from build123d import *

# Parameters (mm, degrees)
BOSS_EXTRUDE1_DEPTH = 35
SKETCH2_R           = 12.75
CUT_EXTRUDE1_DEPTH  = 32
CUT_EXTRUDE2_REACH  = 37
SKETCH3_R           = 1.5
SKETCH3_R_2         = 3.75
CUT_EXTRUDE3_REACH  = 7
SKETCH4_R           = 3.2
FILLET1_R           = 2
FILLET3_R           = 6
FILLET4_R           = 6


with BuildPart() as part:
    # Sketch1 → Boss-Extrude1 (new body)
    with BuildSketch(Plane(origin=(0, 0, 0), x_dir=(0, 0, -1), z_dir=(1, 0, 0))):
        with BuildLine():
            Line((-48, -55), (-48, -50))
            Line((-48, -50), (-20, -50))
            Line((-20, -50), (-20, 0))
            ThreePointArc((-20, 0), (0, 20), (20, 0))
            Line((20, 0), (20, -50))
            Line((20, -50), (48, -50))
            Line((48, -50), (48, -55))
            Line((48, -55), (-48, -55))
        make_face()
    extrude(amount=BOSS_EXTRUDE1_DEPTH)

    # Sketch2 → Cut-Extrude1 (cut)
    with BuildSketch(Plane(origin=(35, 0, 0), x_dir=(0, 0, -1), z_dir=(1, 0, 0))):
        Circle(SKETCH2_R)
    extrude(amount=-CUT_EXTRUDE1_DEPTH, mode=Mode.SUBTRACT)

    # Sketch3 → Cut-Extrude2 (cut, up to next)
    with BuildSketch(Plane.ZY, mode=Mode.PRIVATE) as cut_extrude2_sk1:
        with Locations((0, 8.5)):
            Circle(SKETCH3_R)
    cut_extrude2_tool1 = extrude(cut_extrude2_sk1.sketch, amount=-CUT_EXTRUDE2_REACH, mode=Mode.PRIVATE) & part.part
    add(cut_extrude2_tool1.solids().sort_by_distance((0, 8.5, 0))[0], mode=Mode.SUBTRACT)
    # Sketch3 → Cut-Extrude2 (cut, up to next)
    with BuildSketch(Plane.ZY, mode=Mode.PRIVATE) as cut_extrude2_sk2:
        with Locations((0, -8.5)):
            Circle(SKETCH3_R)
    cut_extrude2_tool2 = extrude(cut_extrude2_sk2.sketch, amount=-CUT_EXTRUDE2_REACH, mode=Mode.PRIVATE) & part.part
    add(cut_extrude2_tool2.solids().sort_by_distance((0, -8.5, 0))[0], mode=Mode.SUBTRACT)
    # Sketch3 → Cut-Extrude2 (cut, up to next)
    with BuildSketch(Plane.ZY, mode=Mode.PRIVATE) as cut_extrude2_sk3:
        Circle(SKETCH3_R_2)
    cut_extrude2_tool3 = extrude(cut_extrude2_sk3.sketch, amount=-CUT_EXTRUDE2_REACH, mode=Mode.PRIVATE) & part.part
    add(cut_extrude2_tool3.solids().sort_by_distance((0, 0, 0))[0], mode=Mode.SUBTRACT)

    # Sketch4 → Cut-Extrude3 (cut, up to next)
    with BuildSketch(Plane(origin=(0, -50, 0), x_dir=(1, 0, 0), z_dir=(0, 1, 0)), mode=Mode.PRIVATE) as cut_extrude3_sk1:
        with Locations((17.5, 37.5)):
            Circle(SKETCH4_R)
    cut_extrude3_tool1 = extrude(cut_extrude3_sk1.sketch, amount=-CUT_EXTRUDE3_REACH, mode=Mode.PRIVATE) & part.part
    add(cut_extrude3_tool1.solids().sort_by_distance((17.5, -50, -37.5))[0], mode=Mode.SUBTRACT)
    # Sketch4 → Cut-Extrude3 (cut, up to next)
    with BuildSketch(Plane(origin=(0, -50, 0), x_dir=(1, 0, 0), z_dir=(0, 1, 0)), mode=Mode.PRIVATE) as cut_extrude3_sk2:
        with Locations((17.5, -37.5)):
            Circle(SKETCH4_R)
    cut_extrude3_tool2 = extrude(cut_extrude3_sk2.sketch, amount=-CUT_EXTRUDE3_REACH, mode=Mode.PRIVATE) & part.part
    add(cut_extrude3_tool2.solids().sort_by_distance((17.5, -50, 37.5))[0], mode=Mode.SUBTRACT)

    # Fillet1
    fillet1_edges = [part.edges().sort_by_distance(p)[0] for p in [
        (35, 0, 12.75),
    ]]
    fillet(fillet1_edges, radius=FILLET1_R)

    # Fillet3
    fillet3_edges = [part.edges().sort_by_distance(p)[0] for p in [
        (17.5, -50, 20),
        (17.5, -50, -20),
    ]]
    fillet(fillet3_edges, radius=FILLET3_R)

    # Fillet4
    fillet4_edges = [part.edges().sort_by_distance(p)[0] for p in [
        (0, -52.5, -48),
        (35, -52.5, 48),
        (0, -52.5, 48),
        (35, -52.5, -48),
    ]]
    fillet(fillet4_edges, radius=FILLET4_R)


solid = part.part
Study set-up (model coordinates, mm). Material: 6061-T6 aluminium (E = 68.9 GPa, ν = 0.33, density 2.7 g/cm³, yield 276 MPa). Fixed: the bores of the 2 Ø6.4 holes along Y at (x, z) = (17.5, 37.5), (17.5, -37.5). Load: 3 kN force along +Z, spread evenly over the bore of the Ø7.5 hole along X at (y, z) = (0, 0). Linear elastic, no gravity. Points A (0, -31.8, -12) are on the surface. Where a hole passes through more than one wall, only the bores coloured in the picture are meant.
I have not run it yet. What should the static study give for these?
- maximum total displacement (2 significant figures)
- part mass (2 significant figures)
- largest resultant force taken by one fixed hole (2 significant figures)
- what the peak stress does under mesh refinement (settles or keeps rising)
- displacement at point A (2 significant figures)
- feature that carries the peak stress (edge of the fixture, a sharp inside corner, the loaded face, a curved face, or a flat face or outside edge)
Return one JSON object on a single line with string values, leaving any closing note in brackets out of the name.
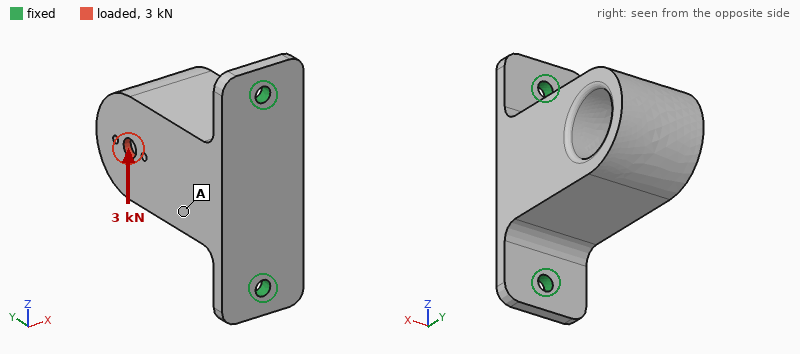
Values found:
{"maximum total displacement": "0.19 mm", "part mass": "250 g", "largest resultant force taken by one fixed hole": "3.1 kN", "what the peak stress does under mesh refinement": "keeps rising", "displacement at point A": "0.057 mm", "feature that carries the peak stress": "edge of the fixture"}
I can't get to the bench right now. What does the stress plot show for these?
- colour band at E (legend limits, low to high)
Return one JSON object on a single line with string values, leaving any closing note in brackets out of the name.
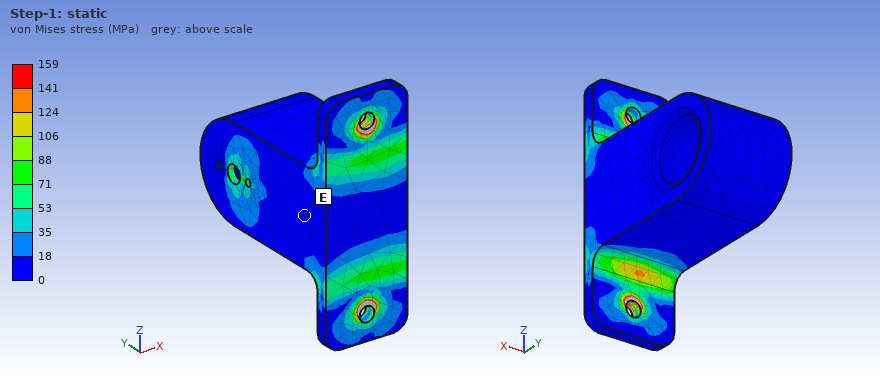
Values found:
{"colour band at E": "0 to 18 MPa"}
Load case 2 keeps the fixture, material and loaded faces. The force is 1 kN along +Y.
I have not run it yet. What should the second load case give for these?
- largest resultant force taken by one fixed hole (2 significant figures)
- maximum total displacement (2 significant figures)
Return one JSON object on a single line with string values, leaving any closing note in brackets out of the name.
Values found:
{"largest resultant force taken by one fixed hole": "590 N", "maximum total displacement": "0.20 mm"}
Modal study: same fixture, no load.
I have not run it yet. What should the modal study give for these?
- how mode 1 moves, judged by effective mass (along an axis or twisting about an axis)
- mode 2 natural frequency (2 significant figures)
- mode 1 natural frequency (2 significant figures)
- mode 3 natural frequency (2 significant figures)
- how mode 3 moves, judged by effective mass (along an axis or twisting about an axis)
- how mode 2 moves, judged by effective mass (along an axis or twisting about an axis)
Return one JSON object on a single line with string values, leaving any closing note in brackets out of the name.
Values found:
{"how mode 1 moves, judged by effective mass": "along X", "mode 2 natural frequency": "2300 Hz", "mode 1 natural frequency": "710 Hz", "mode 3 natural frequency": "3000 Hz", "how mode 3 moves, judged by effective mass": "along Y", "how mode 2 moves, judged by effective mass": "along Z"}
